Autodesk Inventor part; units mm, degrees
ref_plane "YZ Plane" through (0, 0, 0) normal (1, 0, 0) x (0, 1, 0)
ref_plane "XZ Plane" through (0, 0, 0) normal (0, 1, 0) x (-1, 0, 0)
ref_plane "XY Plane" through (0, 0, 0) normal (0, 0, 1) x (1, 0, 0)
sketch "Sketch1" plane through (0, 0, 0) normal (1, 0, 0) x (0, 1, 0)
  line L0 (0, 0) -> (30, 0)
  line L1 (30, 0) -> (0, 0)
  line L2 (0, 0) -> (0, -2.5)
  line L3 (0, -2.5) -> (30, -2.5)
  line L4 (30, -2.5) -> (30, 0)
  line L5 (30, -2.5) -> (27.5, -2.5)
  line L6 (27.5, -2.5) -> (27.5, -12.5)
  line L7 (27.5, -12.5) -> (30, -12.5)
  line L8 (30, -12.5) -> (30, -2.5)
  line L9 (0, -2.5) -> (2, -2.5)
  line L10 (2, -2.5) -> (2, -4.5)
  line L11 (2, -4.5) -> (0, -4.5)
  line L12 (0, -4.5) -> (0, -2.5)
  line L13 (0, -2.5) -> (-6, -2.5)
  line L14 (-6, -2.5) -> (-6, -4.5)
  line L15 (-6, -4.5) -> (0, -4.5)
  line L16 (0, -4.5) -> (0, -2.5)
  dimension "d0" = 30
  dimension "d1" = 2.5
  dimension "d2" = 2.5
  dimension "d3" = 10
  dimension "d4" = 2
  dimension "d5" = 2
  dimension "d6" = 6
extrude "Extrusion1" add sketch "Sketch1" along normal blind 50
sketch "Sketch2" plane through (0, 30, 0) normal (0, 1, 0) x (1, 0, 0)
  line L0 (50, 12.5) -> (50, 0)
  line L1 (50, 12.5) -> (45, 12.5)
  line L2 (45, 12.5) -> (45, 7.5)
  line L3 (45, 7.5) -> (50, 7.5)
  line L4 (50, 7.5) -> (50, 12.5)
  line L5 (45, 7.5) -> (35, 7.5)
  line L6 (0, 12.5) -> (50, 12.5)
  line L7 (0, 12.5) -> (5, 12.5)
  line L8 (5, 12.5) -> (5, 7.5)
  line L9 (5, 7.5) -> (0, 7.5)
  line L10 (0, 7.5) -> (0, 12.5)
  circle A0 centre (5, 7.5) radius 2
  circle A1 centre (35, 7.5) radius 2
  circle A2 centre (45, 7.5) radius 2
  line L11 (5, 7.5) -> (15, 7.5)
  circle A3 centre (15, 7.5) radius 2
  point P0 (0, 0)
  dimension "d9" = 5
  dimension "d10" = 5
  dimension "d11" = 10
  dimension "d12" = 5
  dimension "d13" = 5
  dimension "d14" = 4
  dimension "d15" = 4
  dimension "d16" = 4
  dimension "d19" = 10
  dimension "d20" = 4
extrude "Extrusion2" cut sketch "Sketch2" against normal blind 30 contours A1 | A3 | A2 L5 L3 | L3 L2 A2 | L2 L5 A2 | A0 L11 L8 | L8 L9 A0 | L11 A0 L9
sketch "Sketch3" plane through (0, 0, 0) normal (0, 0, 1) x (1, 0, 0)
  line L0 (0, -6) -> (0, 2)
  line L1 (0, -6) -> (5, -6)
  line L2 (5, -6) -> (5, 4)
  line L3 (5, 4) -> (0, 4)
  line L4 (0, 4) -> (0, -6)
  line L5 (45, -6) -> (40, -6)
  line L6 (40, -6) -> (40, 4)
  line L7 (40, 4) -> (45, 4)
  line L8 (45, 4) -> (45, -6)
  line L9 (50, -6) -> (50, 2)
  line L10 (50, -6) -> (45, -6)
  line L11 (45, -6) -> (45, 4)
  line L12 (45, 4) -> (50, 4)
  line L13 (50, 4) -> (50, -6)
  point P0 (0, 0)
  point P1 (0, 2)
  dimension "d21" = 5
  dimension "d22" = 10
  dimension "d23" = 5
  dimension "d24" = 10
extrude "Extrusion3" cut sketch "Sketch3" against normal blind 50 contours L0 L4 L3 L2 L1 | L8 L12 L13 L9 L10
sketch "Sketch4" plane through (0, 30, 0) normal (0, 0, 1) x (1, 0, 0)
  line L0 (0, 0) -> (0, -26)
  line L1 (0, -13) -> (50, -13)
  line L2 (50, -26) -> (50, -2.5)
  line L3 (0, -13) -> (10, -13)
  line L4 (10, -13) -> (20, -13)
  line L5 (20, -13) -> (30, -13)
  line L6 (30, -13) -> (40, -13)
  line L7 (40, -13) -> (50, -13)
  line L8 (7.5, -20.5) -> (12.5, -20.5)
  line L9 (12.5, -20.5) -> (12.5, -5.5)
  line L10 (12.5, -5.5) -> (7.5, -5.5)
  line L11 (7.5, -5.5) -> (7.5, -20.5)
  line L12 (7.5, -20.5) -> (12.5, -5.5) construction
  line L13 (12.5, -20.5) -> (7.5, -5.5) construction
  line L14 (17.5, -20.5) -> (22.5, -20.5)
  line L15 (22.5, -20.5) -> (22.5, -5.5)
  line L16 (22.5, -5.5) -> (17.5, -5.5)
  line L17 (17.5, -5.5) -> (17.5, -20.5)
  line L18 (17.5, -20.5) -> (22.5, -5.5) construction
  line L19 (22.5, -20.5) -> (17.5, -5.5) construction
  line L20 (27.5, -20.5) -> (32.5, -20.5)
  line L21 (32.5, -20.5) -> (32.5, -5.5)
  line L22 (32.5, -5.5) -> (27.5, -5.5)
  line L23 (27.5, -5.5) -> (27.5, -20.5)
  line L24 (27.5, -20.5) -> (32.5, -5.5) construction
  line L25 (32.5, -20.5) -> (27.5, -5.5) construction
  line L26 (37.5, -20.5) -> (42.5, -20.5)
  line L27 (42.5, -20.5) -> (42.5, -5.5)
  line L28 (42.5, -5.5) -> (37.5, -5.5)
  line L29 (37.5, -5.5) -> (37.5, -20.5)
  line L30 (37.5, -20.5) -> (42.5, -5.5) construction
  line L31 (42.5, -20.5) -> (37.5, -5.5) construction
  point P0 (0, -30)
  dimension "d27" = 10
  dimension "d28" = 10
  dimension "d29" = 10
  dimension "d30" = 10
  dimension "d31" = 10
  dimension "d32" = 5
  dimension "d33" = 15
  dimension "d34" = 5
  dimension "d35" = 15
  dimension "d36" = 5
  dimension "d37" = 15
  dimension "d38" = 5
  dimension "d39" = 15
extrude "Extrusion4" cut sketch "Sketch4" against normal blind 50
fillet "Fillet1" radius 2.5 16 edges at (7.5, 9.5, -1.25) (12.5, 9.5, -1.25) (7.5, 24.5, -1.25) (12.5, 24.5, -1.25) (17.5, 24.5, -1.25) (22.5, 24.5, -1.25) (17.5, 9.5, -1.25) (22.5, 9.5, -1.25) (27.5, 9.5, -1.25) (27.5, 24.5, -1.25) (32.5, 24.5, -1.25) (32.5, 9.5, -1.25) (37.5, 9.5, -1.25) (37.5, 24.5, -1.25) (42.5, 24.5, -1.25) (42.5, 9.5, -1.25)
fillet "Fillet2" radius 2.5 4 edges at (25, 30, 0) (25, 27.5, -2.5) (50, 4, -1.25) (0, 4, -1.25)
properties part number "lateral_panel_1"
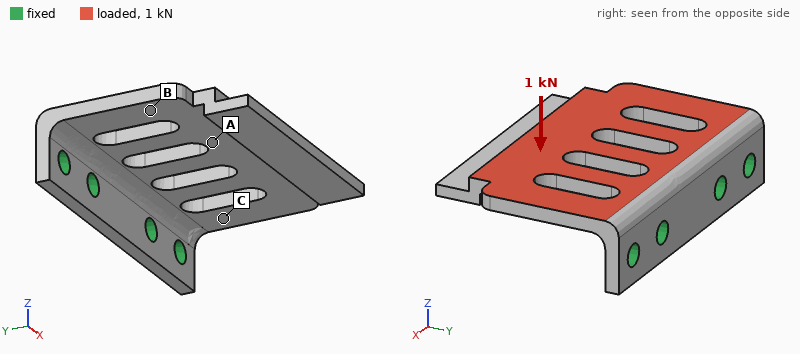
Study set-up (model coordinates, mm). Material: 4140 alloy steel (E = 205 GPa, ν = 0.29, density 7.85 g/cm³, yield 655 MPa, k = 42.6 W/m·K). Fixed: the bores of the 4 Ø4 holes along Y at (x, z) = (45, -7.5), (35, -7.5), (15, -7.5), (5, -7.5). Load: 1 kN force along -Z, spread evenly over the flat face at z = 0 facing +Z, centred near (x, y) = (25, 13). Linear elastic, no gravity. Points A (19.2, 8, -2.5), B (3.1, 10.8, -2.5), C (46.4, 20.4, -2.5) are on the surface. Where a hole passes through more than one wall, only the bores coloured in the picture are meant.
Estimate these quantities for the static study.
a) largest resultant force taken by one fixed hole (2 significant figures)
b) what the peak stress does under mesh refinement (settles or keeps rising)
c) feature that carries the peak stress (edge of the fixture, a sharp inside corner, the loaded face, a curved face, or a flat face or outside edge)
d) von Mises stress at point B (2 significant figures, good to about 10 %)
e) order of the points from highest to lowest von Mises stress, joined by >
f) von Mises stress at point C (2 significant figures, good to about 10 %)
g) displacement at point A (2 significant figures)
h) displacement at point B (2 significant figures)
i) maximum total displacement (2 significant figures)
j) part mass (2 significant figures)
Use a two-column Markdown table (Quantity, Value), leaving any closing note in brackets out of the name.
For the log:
| Quantity | Value |
|---|---|
| largest resultant force taken by one fixed hole | 300 N |
| what the peak stress does under mesh refinement | keeps rising |
| feature that carries the peak stress | edge of the fixture |
| von Mises stress at point B | 74 MPa |
| order of the points from highest to lowest von Mises stress, joined by > | C > B > A |
| von Mises stress at point C | 230 MPa |
| displacement at point A | 0.26 mm |
| displacement at point B | 0.21 mm |
| maximum total displacement | 0.52 mm |
| part mass | 37 g |
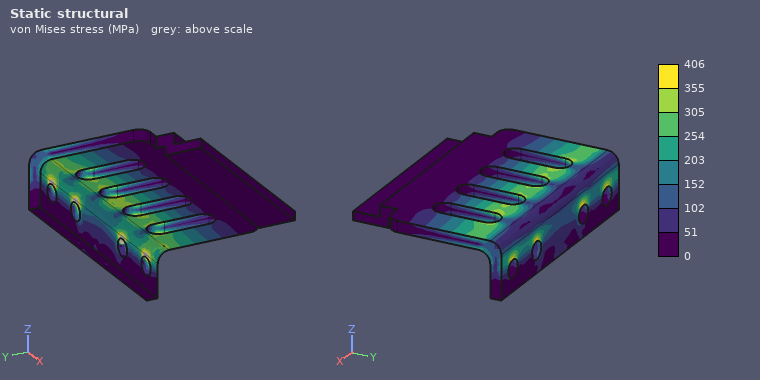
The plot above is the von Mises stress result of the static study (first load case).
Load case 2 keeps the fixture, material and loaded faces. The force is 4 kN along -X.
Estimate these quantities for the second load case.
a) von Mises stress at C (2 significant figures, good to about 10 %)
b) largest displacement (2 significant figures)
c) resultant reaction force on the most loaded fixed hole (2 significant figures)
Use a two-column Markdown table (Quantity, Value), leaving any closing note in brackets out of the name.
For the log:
| Quantity | Value |
|---|---|
| von Mises stress at C | 120 MPa |
| largest displacement | 67 µm |
| resultant reaction force on the most loaded fixed hole | 1.6 kN |
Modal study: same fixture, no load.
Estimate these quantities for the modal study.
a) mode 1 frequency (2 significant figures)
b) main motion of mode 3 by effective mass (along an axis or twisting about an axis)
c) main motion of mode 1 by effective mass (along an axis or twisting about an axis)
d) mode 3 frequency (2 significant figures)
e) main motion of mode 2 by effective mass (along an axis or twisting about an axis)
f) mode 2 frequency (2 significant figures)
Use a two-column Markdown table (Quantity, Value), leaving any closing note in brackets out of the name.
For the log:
| Quantity | Value |
|---|---|
| mode 1 frequency | 1500 Hz |
| main motion of mode 3 by effective mass | along X |
| main motion of mode 1 by effective mass | along Z |
| mode 3 frequency | 7800 Hz |
| main motion of mode 2 by effective mass | twisting about Y |
| mode 2 frequency | 3200 Hz |
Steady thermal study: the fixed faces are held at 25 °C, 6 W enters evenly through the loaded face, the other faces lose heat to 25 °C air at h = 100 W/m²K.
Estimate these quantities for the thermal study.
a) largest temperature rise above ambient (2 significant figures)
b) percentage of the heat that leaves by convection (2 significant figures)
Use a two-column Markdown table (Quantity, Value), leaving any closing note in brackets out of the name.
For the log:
| Quantity | Value |
|---|---|
| largest temperature rise above ambient | 14 K |
| percentage of the heat that leaves by convection | 45 % |
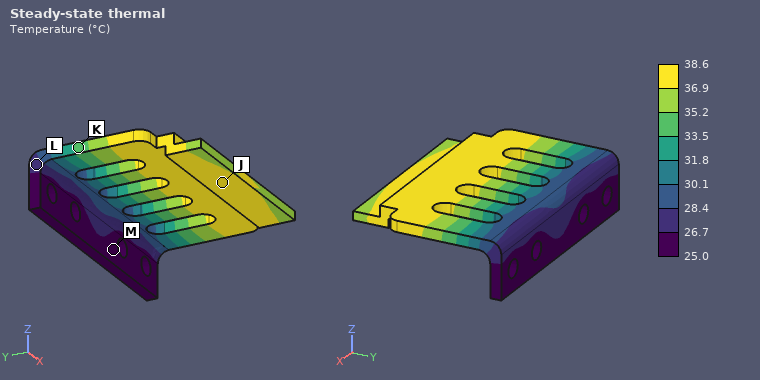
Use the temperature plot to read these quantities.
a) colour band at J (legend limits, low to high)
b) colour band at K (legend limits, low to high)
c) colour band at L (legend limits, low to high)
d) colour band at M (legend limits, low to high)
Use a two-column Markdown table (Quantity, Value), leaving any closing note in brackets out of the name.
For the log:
| Quantity | Value |
|---|---|
| colour band at J | 36.9 to 38.6 °C |
| colour band at K | 33.5 to 35.2 °C |
| colour band at L | 26.7 to 28.4 °C |
| colour band at M | 25.0 to 26.7 °C |
